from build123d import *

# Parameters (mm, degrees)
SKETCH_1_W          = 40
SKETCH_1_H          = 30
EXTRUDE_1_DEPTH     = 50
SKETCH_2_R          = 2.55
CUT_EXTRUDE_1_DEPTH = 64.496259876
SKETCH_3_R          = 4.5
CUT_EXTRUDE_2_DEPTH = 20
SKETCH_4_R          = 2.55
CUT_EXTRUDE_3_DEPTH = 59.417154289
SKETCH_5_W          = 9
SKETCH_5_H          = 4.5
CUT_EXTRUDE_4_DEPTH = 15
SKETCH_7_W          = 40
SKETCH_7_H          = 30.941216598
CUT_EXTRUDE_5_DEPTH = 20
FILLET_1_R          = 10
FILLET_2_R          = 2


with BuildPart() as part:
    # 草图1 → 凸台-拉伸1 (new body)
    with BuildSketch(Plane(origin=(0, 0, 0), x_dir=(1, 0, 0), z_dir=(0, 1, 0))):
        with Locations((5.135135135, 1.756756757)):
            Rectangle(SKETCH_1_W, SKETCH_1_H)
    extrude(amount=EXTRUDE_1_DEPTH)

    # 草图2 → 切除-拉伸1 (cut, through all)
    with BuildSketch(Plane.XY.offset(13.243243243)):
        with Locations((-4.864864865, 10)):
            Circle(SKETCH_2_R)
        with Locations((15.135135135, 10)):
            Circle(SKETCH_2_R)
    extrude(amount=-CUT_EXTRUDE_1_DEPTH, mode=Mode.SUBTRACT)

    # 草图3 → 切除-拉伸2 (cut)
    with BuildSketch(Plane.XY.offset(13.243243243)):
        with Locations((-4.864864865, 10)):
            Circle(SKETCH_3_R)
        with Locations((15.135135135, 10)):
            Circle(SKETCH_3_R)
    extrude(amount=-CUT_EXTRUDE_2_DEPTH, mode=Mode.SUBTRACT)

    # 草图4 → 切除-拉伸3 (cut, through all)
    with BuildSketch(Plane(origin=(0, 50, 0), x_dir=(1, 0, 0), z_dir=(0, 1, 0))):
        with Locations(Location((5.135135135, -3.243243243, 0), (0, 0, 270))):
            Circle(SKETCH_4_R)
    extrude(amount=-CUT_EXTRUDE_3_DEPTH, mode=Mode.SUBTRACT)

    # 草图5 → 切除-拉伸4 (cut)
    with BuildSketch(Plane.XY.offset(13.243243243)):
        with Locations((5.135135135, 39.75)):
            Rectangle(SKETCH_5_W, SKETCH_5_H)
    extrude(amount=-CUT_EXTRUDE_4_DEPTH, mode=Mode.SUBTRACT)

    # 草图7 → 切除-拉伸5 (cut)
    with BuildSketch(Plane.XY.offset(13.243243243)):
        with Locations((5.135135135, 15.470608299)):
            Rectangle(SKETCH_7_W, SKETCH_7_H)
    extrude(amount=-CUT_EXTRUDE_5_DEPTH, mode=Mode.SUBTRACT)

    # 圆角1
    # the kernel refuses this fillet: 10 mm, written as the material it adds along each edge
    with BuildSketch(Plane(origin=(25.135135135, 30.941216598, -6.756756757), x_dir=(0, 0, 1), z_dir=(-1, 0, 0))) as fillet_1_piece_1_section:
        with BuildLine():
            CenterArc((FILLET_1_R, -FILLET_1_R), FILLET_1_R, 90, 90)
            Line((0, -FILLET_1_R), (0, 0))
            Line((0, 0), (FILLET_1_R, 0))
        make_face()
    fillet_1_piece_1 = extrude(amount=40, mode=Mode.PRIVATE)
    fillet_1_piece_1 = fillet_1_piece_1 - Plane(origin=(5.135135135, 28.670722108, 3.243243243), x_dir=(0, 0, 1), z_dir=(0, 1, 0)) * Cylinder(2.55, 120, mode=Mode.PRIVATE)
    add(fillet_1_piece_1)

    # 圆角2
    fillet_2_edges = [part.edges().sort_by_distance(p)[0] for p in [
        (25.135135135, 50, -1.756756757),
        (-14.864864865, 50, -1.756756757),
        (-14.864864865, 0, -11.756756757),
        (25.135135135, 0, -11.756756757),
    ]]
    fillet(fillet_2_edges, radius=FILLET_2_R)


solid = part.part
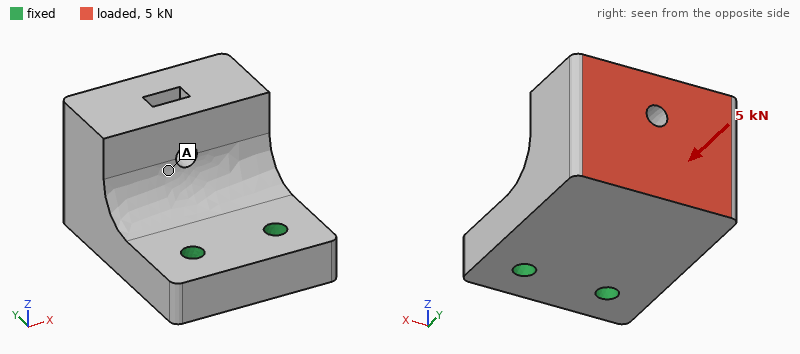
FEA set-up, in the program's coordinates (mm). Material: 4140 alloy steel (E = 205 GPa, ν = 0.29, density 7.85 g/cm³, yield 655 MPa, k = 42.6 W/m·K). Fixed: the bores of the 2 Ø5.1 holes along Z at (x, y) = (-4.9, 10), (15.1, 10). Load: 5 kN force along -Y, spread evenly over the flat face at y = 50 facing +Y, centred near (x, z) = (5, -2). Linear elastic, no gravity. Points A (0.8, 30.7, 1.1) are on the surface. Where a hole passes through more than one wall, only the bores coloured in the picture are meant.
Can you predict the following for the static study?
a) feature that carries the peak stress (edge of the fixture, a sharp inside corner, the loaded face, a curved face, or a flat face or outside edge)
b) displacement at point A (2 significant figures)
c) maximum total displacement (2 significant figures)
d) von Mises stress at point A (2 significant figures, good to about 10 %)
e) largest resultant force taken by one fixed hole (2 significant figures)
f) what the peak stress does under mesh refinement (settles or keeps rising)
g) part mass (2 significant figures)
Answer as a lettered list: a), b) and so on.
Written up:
a) edge of the fixture
b) 25 µm
c) 57 µm
d) 17 MPa
e) 2.5 kN
f) keeps rising
g) 270 g
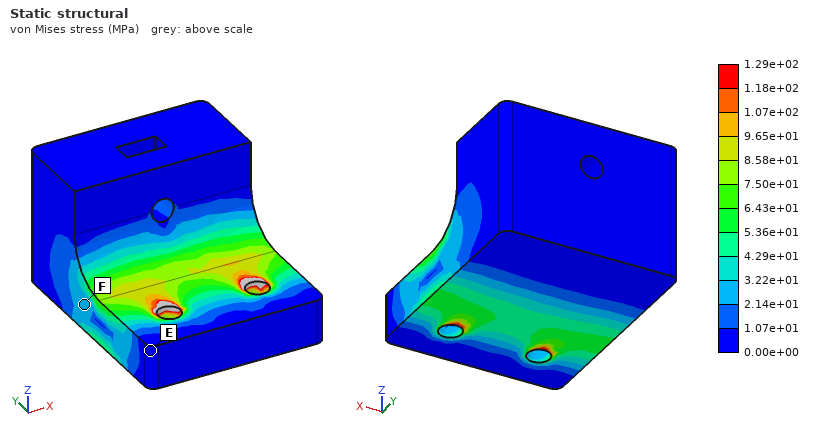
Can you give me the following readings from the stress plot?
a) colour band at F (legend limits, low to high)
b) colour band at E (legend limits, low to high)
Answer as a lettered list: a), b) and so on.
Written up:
a) 2.14e+01 to 3.22e+01 MPa
b) 0.00e+00 to 1.07e+01 MPa
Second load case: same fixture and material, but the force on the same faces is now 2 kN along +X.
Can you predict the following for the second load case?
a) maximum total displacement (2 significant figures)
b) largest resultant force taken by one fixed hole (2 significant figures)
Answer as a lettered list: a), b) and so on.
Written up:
a) 12 µm
b) 3.6 kN
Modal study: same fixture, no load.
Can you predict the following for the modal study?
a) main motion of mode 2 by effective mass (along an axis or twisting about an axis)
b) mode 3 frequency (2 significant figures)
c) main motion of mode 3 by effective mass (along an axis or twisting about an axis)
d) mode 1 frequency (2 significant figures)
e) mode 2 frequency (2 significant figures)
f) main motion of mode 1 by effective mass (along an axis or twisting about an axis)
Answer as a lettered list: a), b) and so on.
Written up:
a) along X
b) 8800 Hz
c) along X
d) 2700 Hz
e) 5700 Hz
f) along Z
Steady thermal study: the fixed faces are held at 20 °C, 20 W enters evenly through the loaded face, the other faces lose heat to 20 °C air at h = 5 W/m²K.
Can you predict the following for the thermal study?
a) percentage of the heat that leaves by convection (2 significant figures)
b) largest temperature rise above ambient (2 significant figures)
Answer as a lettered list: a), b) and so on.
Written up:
a) 3.7 %
b) 36 K
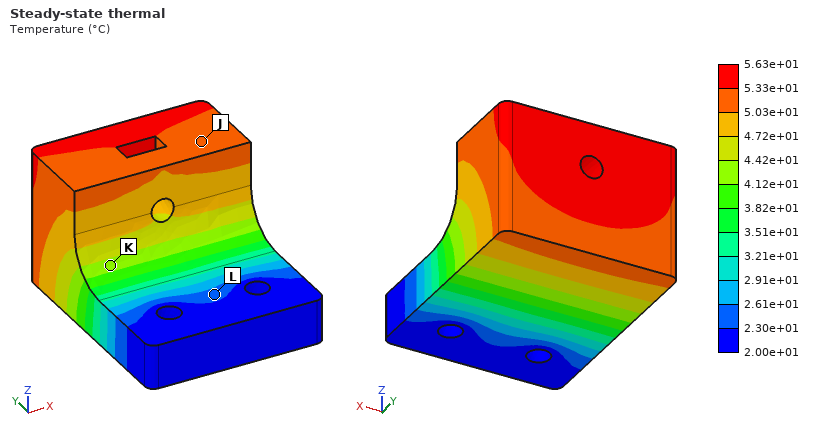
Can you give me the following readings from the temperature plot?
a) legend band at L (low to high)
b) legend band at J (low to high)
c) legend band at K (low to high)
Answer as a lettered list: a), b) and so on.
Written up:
a) 2.30e+01 to 2.61e+01 °C
b) 5.03e+01 to 5.33e+01 °C
c) 4.12e+01 to 4.42e+01 °C
